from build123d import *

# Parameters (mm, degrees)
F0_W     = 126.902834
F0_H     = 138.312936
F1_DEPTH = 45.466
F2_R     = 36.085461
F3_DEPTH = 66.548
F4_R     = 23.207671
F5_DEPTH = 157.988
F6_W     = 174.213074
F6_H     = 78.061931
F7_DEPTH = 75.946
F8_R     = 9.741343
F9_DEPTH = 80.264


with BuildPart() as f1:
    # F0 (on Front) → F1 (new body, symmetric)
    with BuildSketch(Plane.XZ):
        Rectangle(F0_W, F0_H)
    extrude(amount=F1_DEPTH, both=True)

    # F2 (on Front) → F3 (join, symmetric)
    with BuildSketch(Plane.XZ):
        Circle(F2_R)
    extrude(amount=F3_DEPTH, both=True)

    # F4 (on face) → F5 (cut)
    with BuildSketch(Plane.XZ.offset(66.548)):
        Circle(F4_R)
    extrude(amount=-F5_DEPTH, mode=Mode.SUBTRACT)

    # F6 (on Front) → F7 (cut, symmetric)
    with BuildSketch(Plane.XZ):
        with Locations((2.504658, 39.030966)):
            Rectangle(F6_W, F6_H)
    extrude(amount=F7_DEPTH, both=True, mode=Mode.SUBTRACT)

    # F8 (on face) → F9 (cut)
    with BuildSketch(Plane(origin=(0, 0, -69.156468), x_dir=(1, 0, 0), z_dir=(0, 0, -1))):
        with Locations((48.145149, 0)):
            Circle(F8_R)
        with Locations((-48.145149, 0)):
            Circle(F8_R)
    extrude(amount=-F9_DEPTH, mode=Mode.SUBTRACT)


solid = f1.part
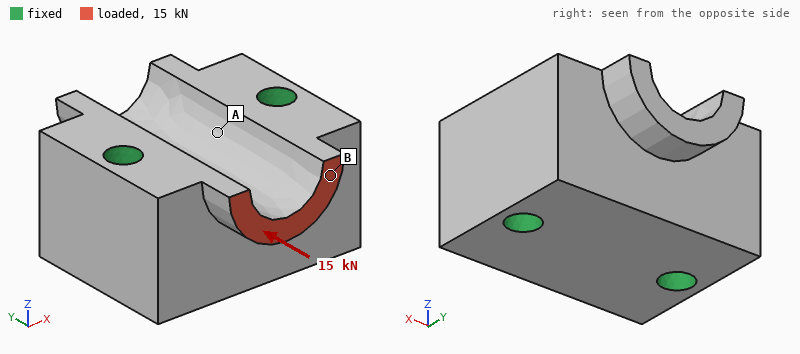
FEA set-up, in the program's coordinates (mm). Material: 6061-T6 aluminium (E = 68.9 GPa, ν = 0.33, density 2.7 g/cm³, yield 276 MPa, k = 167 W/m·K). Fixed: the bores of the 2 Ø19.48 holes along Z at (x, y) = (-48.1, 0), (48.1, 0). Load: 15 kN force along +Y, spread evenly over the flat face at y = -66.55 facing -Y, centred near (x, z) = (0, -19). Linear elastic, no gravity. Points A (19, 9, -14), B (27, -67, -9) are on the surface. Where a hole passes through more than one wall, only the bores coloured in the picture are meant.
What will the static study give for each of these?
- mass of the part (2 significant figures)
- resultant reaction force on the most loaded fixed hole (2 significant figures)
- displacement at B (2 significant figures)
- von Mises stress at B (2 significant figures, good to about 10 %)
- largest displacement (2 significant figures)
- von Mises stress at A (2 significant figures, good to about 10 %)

2.0 kg
7.8 kN
11 µm
13 MPa
13 µm
2.1 MPa
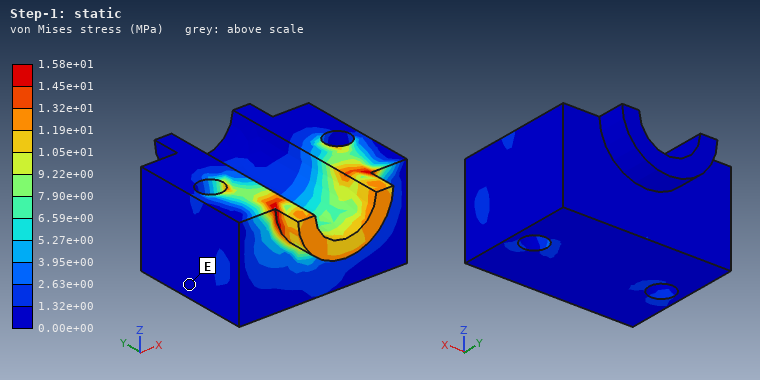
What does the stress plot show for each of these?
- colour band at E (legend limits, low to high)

0.00e+00 to 1.32e+00 MPa
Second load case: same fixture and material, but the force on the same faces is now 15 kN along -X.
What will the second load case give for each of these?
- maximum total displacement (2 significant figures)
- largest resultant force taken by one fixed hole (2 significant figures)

72 µm
12 kN
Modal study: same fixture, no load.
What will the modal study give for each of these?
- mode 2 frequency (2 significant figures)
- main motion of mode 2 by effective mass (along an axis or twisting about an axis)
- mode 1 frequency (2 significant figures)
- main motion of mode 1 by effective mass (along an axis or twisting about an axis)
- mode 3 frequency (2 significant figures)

11 kHz
along Z
10 kHz
twisting about X
12 kHz
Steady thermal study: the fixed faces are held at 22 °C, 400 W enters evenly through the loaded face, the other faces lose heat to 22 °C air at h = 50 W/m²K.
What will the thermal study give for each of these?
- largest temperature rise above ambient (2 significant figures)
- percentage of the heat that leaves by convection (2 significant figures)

72 K
5.7 %
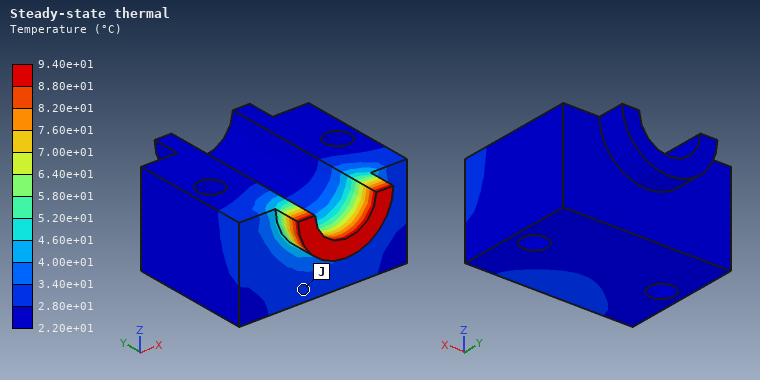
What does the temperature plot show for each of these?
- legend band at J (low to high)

2.80e+01 to 3.40e+01 °C
